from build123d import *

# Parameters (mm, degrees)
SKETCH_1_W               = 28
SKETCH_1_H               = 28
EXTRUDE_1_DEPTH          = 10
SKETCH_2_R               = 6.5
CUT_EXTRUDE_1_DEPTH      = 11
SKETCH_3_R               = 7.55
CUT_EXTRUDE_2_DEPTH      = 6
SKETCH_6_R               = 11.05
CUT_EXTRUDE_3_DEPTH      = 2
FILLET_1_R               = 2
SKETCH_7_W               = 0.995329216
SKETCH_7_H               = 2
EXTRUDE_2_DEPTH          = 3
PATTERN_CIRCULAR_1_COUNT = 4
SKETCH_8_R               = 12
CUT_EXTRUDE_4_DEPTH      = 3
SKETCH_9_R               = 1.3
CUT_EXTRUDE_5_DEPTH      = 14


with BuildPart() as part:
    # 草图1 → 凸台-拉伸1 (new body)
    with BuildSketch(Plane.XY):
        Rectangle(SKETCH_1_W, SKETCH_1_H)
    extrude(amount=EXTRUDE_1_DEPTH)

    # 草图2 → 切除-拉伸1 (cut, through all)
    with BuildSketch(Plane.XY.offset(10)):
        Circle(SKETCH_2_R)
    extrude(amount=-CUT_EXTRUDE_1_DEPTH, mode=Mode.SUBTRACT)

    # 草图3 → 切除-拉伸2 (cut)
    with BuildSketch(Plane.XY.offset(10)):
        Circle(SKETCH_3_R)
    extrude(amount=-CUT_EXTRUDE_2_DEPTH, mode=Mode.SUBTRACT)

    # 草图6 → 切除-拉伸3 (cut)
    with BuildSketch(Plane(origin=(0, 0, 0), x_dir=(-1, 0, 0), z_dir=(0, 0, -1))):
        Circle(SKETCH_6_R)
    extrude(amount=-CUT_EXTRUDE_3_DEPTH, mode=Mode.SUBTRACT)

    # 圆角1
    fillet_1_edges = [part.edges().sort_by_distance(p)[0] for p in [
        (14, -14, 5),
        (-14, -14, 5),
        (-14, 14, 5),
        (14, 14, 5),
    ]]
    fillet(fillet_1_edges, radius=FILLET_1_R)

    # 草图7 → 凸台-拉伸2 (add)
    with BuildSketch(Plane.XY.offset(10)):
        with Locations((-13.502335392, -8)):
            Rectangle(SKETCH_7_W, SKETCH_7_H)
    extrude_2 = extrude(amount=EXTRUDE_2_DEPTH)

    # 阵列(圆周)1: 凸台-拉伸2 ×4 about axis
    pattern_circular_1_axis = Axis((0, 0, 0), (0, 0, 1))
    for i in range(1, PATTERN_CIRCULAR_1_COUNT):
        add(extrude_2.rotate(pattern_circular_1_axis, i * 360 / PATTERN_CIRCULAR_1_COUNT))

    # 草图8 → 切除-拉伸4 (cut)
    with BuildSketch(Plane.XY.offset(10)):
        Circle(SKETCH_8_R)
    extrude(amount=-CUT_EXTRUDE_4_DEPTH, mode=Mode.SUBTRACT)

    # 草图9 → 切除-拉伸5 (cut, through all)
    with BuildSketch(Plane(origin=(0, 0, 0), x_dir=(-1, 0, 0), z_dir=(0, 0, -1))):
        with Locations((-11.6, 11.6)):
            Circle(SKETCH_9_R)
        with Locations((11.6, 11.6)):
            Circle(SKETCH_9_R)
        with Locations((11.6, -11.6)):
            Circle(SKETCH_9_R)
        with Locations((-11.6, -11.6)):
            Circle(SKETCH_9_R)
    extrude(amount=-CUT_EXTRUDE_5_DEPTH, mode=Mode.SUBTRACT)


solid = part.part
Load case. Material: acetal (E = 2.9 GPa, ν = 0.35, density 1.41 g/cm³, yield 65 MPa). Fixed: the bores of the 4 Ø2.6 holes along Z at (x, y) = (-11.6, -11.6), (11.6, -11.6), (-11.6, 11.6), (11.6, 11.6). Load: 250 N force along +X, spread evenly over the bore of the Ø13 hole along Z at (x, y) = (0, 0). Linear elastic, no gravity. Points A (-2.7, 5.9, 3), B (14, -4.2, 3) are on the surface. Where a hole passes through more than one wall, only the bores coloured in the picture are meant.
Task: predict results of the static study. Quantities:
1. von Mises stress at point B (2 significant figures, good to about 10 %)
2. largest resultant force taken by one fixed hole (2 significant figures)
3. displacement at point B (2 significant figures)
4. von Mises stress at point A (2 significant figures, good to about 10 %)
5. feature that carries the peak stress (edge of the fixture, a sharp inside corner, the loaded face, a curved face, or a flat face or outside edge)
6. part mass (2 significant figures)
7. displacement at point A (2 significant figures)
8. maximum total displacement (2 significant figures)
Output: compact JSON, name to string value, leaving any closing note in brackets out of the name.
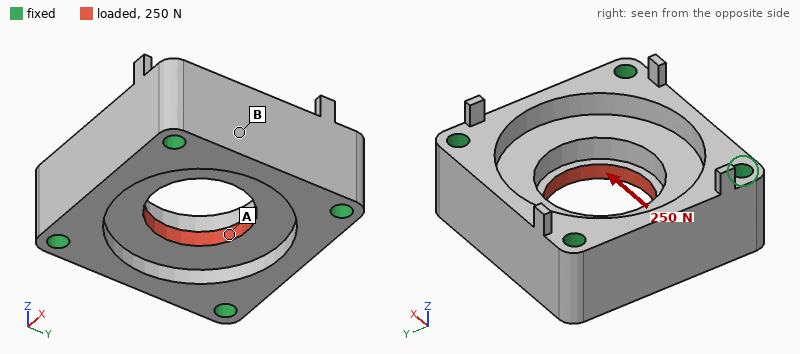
{"von Mises stress at point B": "0.93 MPa", "largest resultant force taken by one fixed hole": "67 N", "displacement at point B": "7.2 µm", "von Mises stress at point A": "5.1 MPa", "feature that carries the peak stress": "a sharp inside corner", "part mass": "6.6 g", "displacement at point A": "8.6 µm", "maximum total displacement": "15 µm"}
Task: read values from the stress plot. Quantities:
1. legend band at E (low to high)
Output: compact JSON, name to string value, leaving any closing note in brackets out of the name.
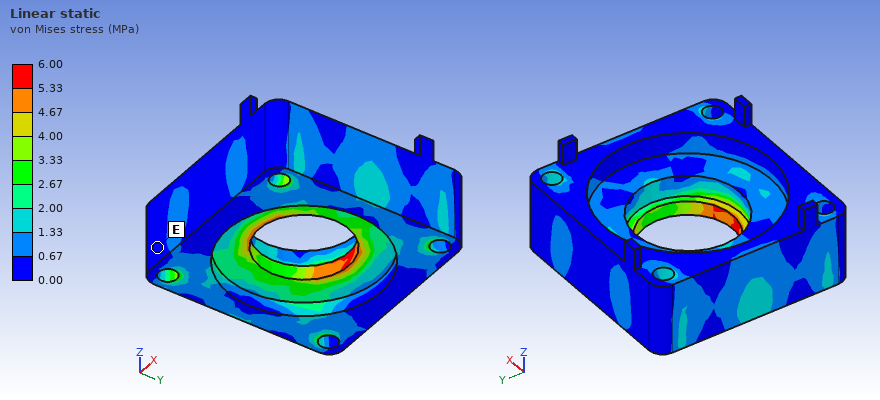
{"legend band at E": "0.00 to 0.67 MPa"}
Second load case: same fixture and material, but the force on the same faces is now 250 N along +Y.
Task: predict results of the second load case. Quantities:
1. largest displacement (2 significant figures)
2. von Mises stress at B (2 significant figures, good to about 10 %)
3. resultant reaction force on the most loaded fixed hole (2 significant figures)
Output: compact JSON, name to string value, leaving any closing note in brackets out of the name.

{"largest displacement": "15 µm", "von Mises stress at B": "0.69 MPa", "resultant reaction force on the most loaded fixed hole": "67 N"}
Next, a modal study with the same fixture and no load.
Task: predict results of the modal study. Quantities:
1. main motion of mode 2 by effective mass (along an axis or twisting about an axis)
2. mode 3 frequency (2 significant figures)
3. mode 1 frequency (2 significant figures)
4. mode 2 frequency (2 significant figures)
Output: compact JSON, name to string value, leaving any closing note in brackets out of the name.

{"main motion of mode 2 by effective mass": "along Z", "mode 3 frequency": "16 kHz", "mode 1 frequency": "11 kHz", "mode 2 frequency": "14 kHz"}
